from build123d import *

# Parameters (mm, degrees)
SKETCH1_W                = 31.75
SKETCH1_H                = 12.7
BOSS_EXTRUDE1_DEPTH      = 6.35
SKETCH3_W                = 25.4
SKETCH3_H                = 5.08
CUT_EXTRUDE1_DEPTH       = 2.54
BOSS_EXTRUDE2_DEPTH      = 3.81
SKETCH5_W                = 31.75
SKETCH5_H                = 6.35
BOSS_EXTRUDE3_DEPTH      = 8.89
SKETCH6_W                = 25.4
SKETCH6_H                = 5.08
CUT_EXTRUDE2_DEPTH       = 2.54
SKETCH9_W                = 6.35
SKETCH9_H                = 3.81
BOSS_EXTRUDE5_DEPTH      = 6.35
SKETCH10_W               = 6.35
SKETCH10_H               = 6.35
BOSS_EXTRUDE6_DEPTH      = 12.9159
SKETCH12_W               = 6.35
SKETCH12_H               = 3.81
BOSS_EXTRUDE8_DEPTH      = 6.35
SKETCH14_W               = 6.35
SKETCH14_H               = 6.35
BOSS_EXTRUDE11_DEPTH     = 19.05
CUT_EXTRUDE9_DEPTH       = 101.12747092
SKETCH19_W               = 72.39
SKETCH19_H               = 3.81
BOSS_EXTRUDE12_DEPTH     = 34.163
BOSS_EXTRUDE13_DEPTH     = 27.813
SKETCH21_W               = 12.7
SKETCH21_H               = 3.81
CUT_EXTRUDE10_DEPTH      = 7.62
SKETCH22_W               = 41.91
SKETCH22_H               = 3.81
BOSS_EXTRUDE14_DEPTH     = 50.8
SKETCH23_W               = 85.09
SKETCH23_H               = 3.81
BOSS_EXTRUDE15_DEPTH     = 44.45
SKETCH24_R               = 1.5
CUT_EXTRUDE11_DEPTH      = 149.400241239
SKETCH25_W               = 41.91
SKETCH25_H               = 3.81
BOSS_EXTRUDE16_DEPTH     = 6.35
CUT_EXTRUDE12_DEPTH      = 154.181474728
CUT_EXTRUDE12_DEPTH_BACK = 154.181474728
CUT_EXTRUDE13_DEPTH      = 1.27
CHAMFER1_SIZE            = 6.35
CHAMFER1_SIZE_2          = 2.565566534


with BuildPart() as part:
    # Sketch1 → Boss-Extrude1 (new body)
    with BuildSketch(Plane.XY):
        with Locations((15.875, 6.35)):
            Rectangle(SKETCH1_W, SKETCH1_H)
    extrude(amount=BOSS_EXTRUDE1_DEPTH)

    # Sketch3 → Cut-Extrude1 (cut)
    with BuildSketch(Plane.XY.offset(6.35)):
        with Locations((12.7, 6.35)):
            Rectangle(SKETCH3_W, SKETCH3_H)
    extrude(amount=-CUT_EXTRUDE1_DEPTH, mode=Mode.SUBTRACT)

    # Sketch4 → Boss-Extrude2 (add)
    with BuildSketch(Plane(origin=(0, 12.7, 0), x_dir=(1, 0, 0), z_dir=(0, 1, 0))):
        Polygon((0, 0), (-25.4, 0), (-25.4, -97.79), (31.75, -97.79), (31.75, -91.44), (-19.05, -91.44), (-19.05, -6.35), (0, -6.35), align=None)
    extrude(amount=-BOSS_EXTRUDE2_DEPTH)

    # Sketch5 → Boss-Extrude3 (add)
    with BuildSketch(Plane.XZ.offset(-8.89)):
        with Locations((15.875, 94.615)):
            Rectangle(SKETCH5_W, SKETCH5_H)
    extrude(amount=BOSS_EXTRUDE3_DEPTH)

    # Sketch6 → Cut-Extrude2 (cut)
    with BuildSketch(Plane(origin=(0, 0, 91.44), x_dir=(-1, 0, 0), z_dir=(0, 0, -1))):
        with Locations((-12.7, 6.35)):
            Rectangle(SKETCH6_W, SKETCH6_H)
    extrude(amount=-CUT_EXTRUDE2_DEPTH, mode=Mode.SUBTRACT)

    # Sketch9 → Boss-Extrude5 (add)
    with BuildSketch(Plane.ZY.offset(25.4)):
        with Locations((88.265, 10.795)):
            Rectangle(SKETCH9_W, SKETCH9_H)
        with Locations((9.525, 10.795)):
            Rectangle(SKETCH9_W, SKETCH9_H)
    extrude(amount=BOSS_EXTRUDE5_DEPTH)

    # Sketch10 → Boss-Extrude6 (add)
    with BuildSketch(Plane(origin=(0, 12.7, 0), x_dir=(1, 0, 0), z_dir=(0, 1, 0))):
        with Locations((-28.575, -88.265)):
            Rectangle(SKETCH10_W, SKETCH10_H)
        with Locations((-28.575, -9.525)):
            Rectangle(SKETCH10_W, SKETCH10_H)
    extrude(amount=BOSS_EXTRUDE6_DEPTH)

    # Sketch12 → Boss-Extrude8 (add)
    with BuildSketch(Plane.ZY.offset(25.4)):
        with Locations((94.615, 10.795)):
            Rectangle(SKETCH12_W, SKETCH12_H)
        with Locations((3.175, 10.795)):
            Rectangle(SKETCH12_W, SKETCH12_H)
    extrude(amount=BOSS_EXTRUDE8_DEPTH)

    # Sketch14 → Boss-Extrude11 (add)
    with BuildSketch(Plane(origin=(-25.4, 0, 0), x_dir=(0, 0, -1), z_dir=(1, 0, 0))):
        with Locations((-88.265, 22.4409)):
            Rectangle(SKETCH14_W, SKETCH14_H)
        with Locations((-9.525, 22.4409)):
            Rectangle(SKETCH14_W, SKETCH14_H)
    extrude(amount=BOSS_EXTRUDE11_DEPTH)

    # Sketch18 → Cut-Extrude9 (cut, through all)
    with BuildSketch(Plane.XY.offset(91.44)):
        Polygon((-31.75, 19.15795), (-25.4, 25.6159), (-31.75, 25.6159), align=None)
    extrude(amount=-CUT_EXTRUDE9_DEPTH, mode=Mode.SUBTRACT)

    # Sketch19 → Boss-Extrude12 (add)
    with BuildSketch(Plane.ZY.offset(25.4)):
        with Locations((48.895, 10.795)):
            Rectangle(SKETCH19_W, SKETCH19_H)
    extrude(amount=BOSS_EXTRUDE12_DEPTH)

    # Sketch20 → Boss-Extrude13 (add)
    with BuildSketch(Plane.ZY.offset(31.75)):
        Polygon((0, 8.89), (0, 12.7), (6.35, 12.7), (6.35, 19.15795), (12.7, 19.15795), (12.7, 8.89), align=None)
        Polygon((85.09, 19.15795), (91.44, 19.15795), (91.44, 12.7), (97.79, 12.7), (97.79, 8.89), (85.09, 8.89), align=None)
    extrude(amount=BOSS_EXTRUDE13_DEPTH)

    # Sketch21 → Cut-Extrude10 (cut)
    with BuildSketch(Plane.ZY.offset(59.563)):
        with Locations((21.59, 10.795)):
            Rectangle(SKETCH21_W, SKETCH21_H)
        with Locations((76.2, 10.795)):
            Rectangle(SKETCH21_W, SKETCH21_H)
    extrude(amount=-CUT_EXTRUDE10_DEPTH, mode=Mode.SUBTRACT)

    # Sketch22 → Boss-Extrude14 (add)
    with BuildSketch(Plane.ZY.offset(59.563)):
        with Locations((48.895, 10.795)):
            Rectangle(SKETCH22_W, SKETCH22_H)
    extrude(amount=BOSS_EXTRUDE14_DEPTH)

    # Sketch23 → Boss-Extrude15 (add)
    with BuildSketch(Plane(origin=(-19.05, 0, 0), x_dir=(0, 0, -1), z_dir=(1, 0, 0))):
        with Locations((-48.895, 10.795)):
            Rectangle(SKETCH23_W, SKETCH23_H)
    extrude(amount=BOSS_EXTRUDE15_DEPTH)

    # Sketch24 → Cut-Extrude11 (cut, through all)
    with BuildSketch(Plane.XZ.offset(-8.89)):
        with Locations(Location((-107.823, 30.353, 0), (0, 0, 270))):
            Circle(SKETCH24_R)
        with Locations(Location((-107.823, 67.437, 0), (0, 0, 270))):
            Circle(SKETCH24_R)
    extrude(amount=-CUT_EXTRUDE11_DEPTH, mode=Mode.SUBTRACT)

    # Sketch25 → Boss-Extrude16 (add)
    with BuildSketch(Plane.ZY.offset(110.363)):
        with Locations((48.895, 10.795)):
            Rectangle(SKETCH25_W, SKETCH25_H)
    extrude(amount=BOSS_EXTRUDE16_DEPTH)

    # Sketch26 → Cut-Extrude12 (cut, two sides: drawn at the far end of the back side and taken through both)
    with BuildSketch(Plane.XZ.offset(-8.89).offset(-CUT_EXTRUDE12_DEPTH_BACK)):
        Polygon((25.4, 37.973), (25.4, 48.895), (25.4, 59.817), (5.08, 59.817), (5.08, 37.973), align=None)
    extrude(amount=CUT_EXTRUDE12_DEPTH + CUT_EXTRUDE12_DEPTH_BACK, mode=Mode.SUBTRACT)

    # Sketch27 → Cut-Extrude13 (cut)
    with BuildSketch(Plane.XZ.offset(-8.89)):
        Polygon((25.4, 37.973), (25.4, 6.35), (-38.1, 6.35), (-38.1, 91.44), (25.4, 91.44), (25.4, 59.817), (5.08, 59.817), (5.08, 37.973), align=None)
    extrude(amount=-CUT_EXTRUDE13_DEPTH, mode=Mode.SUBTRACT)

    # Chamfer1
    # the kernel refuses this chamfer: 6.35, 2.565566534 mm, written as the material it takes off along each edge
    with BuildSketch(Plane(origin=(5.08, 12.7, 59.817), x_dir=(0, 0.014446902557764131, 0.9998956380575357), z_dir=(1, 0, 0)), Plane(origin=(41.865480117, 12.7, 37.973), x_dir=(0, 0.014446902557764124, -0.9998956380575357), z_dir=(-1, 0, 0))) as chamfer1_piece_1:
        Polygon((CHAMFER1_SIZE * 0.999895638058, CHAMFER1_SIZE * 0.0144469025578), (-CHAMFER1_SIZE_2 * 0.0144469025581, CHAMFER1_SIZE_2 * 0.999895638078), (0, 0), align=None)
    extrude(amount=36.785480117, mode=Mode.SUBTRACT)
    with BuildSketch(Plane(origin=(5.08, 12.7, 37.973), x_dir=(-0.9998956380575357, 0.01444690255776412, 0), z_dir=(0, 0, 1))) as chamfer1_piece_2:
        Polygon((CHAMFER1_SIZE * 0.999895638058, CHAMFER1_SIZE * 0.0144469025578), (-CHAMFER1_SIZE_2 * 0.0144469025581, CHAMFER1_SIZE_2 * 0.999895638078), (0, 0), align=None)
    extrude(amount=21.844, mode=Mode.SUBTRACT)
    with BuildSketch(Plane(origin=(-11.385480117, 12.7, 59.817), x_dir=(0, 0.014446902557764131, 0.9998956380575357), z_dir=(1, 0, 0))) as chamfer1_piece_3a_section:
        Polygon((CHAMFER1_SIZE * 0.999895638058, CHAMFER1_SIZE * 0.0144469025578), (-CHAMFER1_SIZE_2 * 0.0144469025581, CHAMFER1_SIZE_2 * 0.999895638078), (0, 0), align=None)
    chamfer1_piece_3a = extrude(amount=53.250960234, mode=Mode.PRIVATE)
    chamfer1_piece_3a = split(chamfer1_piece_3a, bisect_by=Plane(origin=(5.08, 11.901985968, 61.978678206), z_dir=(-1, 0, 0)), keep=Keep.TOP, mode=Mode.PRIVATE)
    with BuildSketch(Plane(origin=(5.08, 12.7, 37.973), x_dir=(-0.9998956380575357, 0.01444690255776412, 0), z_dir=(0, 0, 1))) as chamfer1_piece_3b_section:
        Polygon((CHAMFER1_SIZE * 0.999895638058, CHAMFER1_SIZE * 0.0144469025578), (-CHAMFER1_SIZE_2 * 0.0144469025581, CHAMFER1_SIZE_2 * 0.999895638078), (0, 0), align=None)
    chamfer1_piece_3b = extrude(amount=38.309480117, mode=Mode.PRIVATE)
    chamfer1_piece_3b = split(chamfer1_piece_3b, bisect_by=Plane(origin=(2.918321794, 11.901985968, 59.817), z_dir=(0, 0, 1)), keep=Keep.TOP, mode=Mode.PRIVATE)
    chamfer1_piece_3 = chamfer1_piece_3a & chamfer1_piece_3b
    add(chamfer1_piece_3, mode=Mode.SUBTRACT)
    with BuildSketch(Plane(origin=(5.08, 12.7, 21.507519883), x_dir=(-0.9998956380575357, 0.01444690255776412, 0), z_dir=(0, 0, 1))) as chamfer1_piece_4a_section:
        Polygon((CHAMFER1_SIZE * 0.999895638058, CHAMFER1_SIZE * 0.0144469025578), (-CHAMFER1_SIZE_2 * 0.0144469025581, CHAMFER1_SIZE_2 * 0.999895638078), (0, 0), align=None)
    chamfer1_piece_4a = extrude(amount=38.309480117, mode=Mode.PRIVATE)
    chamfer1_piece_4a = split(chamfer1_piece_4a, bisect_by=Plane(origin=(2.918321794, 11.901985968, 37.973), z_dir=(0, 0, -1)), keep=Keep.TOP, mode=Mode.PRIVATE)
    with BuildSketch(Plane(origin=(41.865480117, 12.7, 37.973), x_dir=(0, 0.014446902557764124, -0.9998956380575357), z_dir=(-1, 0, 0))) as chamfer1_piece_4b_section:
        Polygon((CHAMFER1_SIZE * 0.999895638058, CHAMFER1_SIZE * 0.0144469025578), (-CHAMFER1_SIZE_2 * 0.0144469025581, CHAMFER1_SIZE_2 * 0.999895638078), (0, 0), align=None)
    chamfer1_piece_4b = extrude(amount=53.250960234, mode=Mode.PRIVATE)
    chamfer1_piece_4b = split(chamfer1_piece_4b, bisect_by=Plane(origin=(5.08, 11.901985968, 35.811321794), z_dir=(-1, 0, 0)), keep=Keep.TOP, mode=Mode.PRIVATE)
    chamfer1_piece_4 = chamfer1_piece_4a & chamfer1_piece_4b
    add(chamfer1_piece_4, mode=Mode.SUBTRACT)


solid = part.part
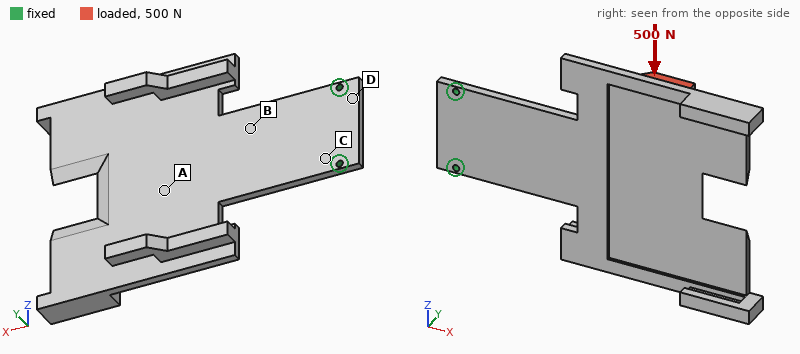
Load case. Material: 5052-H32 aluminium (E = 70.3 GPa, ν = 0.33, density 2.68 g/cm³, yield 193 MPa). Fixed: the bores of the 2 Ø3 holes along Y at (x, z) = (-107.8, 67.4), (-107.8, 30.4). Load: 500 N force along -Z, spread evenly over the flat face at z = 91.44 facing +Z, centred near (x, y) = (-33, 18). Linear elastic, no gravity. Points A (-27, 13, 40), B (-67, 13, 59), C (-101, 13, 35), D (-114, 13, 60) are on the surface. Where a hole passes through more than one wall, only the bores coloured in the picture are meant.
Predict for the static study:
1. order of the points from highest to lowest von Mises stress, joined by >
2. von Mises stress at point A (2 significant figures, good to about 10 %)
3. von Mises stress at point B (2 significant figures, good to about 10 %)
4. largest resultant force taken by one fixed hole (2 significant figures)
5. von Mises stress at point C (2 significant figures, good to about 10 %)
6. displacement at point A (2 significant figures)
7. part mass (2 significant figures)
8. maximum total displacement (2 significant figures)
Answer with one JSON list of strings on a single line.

["B > C > A > D", "16 MPa", "45 MPa", "1.0 kN", "28 MPa", "0.15 mm", "110 g", "0.85 mm"]
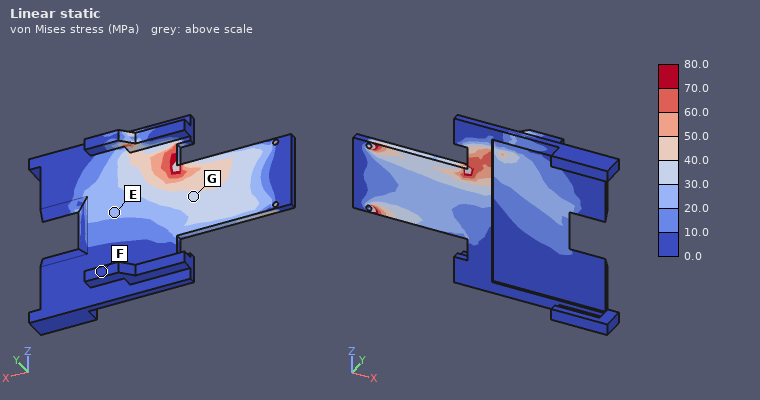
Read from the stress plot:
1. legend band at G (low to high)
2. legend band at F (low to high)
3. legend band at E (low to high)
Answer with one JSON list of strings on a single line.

["30.0 to 40.0 MPa", "0.0 to 10.0 MPa", "20.0 to 30.0 MPa"]
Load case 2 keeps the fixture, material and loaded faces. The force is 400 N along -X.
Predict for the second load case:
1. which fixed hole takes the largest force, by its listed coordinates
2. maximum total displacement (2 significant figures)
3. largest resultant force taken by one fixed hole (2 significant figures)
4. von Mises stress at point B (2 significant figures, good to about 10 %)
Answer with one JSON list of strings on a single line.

["(-107.8, 67.4)", "2.1 mm", "660 N", "43 MPa"]
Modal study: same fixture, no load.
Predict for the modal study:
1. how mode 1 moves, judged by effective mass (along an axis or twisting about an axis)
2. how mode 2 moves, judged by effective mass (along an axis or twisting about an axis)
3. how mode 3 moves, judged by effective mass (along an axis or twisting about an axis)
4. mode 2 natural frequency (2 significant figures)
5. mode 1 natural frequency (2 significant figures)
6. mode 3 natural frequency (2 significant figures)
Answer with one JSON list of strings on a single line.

["along Y", "twisting about X", "along Y", "260 Hz", "120 Hz", "680 Hz"]
